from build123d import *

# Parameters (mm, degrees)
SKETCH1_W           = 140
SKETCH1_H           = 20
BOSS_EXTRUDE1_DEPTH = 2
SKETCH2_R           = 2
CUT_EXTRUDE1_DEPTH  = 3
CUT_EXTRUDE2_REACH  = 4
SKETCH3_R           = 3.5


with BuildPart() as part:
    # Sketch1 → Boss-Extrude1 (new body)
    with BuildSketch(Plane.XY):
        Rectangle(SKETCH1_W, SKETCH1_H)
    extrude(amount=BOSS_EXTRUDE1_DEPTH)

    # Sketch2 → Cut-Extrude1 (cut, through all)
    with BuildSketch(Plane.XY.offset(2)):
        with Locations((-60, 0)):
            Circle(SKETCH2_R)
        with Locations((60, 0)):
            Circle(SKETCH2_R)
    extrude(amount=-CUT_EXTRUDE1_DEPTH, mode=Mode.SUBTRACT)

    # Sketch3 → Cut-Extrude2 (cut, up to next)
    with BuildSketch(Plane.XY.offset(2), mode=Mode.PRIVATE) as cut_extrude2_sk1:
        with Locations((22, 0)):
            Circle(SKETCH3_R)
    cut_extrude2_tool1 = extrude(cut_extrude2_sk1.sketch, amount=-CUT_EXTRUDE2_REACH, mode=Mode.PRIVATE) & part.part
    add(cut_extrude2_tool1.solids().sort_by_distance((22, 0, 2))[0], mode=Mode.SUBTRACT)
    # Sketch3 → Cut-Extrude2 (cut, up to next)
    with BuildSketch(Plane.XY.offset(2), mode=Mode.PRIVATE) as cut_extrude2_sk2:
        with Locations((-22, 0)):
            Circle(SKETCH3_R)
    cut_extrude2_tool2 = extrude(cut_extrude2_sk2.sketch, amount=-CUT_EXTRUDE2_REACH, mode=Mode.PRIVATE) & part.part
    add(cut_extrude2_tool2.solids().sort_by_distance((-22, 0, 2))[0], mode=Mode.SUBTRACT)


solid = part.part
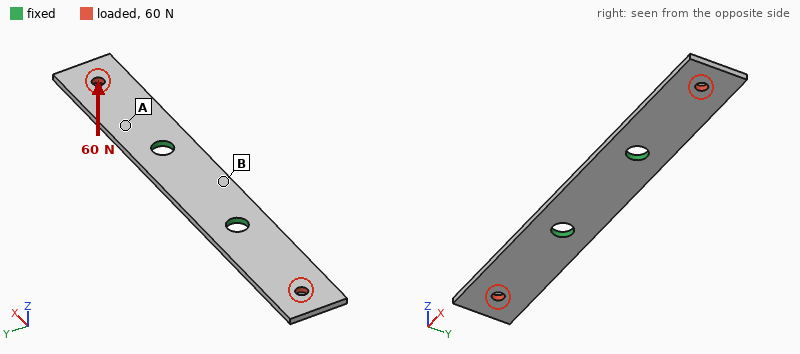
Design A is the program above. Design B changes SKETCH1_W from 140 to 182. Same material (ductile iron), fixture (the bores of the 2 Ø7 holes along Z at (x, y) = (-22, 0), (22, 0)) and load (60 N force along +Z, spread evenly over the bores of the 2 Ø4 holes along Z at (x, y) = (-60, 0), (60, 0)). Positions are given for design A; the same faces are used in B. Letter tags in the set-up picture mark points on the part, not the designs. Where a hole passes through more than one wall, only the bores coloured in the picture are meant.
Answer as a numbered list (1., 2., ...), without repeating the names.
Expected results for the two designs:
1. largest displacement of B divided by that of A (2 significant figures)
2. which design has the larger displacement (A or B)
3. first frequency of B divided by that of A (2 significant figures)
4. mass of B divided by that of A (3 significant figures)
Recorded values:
1. 1.6
2. B
3. 0.46
4. 1.31
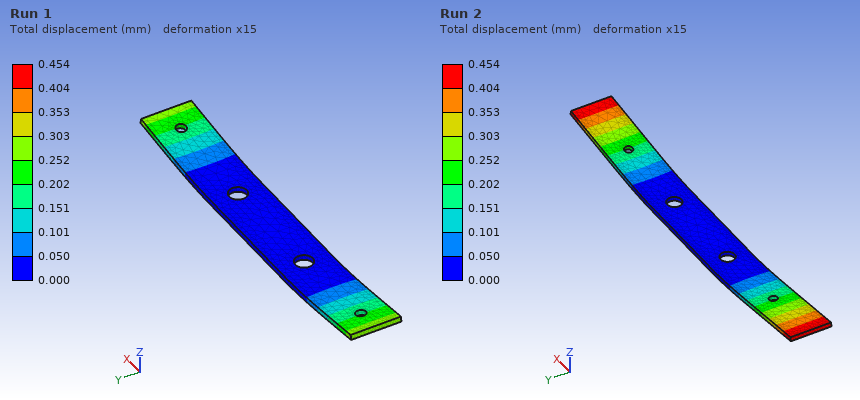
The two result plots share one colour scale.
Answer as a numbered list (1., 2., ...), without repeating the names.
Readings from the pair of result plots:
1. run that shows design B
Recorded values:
1. Run 2
